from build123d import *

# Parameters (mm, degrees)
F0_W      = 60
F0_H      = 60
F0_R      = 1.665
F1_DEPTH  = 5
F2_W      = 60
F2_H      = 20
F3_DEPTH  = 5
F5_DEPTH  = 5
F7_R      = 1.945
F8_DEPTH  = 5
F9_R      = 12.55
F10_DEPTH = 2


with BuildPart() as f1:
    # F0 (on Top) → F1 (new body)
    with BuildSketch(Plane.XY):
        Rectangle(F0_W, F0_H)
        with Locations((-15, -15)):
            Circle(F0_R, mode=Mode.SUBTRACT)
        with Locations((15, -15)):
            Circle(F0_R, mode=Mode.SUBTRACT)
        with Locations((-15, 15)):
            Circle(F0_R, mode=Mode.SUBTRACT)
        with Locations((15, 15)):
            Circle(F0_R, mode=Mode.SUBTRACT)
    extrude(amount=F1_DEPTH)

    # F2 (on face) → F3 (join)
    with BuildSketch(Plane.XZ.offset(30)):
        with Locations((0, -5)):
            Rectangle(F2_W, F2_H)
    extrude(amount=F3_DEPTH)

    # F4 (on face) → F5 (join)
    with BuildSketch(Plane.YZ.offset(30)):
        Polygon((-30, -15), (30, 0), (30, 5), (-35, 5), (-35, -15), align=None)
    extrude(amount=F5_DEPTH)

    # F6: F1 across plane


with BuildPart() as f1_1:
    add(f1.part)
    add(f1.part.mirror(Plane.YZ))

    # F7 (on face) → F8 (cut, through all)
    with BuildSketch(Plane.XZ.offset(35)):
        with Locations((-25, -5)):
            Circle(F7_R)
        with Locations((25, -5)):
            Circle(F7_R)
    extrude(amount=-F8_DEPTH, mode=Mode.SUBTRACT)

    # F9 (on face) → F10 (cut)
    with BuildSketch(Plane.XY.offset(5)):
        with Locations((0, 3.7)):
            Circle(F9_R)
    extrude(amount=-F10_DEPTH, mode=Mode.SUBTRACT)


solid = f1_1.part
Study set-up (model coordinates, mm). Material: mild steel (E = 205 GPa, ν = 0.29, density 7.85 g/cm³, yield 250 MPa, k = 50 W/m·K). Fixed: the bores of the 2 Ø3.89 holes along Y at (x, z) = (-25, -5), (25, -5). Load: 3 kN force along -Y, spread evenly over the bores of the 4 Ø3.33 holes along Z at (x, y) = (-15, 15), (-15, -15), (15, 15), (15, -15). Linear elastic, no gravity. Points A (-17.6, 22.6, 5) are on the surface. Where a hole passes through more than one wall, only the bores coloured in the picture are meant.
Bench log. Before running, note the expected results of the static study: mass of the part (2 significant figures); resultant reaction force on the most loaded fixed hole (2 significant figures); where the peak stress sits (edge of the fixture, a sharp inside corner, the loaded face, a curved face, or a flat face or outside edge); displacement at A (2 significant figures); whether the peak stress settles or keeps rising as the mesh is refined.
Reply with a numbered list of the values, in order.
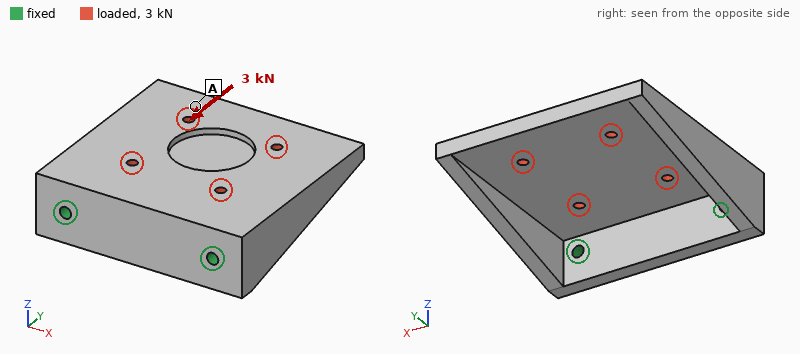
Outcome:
1. 250 g
2. 1.5 kN
3. edge of the fixture
4. 45 µm
5. keeps rising
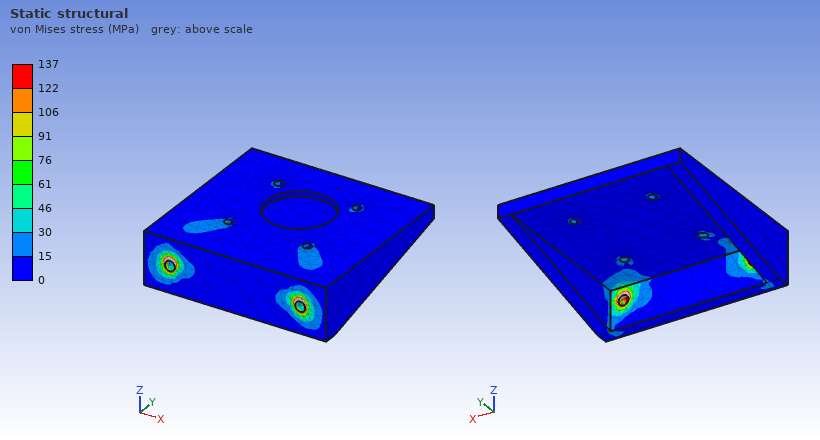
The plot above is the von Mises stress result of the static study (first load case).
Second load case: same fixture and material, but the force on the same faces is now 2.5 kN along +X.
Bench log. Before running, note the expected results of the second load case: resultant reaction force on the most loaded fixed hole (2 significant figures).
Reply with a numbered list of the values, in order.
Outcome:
1. 2.0 kN
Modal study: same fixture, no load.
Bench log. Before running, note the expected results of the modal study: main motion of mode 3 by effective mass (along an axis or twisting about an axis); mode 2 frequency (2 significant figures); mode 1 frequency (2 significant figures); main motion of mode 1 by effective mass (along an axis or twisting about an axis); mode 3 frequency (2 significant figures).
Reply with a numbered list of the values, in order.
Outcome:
1. along X
2. 2600 Hz
3. 1400 Hz
4. along Z
5. 6000 Hz
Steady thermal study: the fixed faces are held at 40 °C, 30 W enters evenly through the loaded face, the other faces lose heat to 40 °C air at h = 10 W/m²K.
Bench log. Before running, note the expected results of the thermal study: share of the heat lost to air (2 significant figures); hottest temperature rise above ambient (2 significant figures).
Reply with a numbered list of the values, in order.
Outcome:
1. 16 %
2. 62 K
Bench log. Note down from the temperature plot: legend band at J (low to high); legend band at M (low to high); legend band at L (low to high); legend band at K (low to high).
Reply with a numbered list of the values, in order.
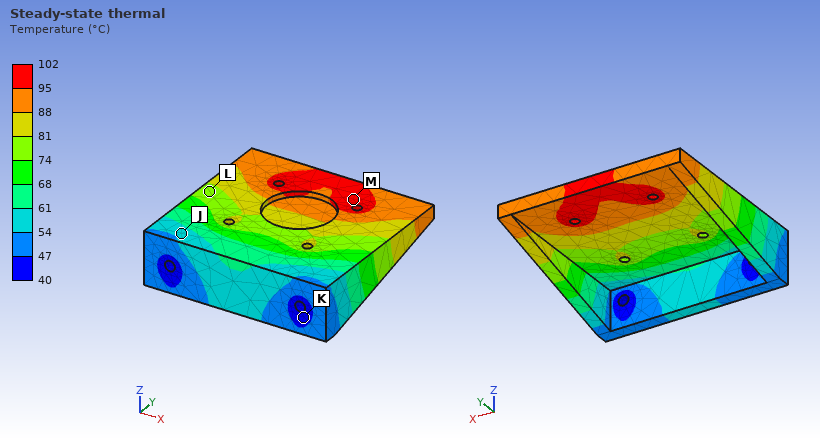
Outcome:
1. 54 to 61 °C
2. 95 to 102 °C
3. 74 to 81 °C
4. 40 to 47 °C
